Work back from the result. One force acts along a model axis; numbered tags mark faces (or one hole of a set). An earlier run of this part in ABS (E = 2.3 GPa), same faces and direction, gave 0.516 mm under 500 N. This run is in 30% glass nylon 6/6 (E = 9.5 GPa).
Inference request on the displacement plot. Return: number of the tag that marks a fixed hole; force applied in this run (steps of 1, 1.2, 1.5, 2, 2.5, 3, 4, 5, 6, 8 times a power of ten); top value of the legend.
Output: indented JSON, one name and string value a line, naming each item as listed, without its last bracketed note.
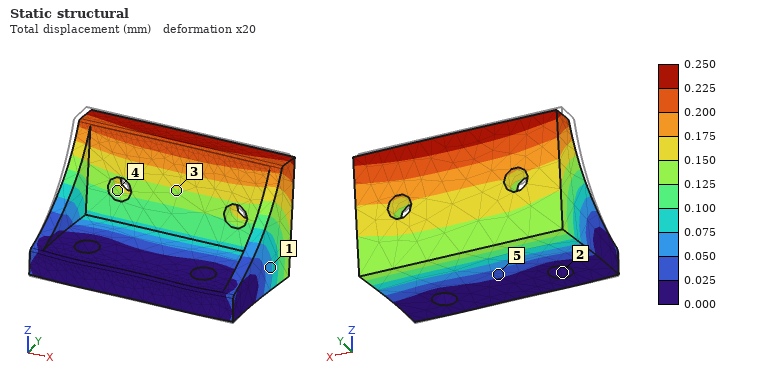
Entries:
{
  "number of the tag that marks a fixed hole": "2",
  "force applied in this run": "1 kN",
  "top value of the legend": "0.250 mm"
}
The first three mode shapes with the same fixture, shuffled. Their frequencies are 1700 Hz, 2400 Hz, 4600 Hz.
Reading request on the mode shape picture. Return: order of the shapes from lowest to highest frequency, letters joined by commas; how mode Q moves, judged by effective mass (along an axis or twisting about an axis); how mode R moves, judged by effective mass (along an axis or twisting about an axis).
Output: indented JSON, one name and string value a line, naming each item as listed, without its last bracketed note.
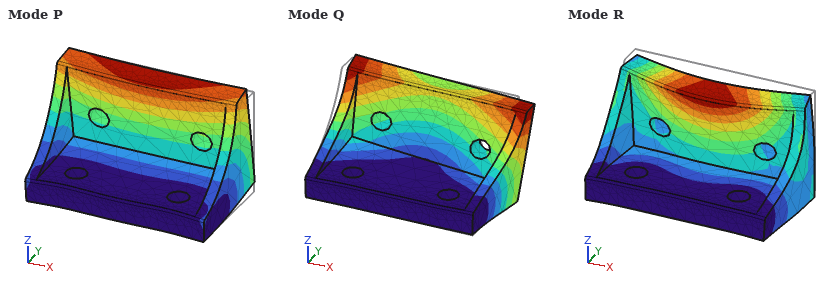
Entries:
{
  "order of the shapes from lowest to highest frequency, letters joined by commas": "P, Q, R",
  "how mode Q moves, judged by effective mass": "along X",
  "how mode R moves, judged by effective mass": "along Z"
}
